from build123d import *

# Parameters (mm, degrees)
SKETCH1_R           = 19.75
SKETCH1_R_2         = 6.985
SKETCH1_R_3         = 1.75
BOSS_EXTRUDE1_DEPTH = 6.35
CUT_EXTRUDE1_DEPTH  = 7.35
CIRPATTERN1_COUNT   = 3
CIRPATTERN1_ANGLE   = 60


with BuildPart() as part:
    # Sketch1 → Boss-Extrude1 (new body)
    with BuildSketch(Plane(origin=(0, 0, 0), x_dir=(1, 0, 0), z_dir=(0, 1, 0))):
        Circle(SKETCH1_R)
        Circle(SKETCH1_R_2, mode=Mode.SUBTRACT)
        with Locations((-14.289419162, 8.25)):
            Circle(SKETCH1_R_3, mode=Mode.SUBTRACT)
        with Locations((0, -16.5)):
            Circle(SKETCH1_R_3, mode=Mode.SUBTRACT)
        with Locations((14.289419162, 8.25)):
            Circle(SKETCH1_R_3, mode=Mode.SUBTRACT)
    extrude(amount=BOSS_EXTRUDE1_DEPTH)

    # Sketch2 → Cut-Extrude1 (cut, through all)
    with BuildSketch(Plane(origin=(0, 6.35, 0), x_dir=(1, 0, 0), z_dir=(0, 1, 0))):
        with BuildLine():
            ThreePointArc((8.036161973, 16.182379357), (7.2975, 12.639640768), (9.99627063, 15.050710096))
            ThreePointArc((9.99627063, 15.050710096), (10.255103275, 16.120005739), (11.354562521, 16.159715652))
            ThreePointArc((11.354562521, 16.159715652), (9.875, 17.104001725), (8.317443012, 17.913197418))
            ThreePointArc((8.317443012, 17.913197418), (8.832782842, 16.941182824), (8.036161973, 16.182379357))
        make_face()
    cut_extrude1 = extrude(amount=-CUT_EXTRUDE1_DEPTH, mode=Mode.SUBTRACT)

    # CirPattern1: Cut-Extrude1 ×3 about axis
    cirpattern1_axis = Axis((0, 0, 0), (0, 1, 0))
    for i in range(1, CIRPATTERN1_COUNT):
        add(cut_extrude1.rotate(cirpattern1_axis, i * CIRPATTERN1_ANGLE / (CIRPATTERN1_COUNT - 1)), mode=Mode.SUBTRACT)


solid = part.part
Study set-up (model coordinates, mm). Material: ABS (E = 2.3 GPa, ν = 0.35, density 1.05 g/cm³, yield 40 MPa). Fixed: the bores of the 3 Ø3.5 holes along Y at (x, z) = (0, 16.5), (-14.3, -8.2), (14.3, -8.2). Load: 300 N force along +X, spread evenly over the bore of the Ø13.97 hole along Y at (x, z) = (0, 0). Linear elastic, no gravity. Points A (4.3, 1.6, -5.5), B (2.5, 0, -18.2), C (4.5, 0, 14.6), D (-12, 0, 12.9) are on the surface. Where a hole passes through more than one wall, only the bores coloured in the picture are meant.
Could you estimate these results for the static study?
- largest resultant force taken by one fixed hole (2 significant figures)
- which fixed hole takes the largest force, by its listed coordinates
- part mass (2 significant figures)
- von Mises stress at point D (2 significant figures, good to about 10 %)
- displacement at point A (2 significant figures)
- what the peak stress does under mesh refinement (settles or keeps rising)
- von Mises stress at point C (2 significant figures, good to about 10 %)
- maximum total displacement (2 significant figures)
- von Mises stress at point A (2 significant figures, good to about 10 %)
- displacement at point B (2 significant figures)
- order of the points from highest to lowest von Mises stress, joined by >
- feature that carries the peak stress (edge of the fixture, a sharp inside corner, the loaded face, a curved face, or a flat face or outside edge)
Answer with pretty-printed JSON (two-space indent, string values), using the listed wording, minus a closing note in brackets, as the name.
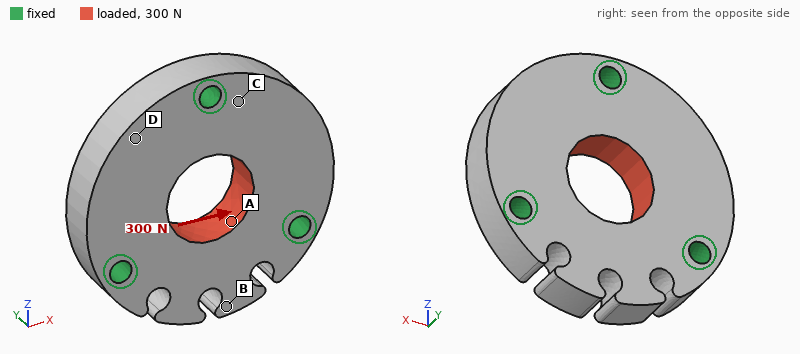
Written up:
{
  "largest resultant force taken by one fixed hole": "110 N",
  "which fixed hole takes the largest force, by its listed coordinates": "(0, 16.5)",
  "part mass": "6.7 g",
  "von Mises stress at point D": "1.00 MPa",
  "displacement at point A": "7.0 µm",
  "what the peak stress does under mesh refinement": "keeps rising",
  "von Mises stress at point C": "1.5 MPa",
  "maximum total displacement": "14 µm",
  "von Mises stress at point A": "2.0 MPa",
  "displacement at point B": "4.7 µm",
  "order of the points from highest to lowest von Mises stress, joined by >": "A > C > D > B",
  "feature that carries the peak stress": "edge of the fixture"
}
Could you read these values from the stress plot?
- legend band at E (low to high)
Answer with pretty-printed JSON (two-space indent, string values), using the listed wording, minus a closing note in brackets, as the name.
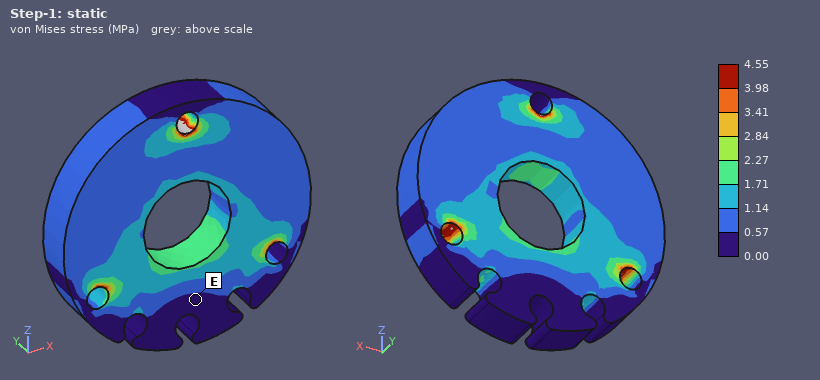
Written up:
{
  "legend band at E": "0.00 to 0.57 MPa"
}
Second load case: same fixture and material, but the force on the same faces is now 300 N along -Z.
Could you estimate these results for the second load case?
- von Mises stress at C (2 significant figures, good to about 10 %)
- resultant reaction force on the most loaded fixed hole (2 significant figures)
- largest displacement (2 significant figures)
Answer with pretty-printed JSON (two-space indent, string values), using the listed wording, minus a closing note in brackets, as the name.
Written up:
{
  "von Mises stress at C": "0.84 MPa",
  "resultant reaction force on the most loaded fixed hole": "100 N",
  "largest displacement": "21 µm"
}
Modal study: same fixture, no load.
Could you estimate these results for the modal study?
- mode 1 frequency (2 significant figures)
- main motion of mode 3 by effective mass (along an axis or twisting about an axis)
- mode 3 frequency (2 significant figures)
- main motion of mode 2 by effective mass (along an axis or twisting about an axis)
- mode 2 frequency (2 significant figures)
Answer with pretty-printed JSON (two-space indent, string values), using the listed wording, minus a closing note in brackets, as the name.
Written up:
{
  "mode 1 frequency": "5900 Hz",
  "main motion of mode 3 by effective mass": "along Y",
  "mode 3 frequency": "7500 Hz",
  "main motion of mode 2 by effective mass": "twisting about Z",
  "mode 2 frequency": "6800 Hz"
}
